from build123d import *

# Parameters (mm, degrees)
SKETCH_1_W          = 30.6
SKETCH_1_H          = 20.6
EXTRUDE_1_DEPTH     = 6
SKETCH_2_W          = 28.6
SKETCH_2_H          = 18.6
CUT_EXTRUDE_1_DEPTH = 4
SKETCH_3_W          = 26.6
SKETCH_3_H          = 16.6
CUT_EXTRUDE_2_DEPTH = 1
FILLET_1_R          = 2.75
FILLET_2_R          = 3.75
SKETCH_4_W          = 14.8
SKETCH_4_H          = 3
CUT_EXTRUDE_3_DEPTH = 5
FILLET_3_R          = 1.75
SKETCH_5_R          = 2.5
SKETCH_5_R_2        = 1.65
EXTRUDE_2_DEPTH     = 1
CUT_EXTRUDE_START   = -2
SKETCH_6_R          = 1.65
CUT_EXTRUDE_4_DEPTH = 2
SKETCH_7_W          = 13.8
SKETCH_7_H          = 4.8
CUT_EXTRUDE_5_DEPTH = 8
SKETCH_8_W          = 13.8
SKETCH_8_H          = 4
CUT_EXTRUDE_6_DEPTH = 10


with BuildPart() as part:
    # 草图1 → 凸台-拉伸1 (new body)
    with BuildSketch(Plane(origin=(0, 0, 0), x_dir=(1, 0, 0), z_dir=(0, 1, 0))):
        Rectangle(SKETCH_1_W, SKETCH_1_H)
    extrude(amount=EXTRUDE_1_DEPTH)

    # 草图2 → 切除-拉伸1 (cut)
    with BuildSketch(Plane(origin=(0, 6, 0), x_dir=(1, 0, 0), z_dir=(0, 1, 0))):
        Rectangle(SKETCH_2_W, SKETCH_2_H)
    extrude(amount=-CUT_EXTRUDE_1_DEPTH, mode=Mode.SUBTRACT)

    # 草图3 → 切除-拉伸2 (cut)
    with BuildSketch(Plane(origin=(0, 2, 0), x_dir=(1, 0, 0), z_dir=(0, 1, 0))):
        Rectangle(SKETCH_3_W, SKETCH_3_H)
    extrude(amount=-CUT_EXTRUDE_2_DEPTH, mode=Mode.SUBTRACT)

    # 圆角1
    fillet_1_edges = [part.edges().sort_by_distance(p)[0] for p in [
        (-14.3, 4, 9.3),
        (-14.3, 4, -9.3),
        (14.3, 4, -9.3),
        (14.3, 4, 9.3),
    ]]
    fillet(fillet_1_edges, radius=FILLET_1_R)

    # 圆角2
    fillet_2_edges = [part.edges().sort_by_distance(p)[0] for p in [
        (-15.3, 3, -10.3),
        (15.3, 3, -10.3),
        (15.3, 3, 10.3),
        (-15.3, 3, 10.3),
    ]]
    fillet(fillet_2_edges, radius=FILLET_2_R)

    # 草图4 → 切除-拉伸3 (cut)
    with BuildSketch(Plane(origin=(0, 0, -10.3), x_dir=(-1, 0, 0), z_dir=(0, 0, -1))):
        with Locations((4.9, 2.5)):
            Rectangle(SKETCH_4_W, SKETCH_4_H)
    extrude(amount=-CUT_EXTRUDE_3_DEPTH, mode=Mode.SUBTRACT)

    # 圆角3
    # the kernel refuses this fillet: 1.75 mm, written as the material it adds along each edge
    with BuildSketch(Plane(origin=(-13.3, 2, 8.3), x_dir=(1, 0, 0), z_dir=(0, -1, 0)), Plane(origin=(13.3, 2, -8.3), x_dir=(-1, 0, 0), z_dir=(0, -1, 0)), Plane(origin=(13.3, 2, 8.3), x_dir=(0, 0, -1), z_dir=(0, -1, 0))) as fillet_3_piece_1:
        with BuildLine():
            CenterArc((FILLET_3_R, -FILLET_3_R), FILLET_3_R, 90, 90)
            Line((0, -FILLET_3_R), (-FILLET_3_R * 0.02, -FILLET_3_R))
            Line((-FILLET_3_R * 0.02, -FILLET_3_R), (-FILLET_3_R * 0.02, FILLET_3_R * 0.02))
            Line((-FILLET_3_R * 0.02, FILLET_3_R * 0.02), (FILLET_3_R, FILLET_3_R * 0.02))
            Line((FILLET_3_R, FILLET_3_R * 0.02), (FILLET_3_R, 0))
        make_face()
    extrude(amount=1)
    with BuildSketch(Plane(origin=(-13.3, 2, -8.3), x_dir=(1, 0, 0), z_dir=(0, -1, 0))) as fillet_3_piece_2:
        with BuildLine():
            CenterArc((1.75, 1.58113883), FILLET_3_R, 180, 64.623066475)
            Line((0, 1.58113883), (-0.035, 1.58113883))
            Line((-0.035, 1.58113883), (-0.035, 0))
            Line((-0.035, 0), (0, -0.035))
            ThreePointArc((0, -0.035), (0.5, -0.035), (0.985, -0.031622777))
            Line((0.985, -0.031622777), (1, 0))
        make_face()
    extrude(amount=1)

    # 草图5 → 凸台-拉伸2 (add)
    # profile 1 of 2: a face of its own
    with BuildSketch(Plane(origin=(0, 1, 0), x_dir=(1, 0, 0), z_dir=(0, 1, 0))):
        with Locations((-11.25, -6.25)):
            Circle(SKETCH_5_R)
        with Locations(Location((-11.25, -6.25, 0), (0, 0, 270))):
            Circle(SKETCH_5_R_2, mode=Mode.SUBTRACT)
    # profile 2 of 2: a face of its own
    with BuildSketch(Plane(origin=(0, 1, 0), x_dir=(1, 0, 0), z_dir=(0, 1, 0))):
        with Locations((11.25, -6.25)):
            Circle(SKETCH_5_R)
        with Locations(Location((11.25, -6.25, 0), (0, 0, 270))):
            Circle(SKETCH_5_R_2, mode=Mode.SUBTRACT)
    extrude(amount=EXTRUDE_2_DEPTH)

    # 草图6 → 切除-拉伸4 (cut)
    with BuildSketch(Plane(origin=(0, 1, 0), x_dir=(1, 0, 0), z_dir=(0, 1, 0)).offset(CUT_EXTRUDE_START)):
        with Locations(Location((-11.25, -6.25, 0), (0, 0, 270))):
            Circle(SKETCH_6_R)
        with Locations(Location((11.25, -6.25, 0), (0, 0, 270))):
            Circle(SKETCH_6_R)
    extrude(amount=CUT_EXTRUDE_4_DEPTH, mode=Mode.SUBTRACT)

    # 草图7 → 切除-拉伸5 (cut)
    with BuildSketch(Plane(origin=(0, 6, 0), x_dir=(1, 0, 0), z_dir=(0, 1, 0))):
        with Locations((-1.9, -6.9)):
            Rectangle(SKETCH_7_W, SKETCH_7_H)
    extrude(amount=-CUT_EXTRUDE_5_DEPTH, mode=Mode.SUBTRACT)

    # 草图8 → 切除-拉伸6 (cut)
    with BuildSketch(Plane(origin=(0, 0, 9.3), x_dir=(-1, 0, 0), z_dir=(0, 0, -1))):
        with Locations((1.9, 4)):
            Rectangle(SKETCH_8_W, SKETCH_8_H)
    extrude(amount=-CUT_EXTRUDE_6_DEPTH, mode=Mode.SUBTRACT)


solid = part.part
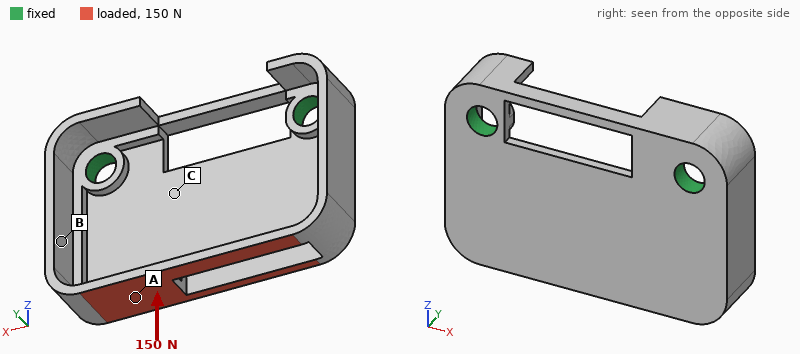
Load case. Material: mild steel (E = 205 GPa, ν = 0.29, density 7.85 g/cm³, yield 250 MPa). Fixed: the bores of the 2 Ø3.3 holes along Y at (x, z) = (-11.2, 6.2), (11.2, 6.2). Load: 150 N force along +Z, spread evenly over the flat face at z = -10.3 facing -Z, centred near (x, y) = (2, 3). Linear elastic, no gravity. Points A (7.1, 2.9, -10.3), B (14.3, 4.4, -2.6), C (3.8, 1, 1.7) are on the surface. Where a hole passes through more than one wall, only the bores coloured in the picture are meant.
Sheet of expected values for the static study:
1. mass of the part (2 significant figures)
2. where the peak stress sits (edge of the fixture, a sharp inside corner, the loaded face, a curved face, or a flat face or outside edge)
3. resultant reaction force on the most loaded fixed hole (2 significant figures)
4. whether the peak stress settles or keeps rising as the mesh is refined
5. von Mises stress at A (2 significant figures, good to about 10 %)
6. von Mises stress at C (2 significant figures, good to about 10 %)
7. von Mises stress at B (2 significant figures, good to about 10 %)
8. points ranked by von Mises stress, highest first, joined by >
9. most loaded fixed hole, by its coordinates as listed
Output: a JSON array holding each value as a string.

["7.7 g", "a sharp inside corner", "94 N", "keeps rising", "63 MPa", "14 MPa", "22 MPa", "A > B > C", "(11.2, 6.2)"]
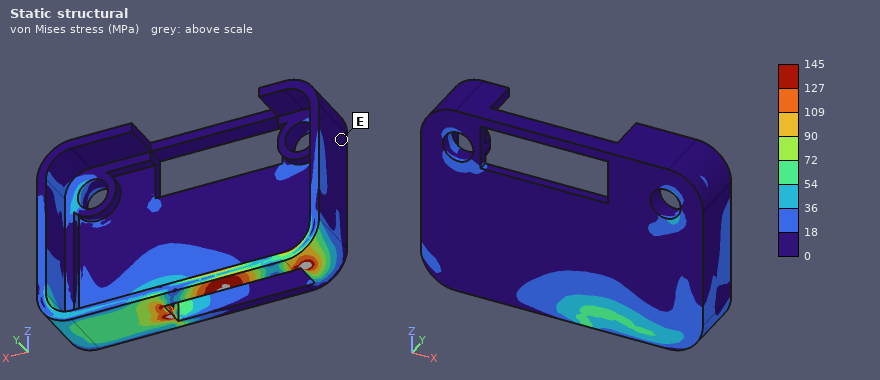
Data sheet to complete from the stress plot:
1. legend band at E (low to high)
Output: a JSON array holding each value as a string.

["0 to 18 MPa"]
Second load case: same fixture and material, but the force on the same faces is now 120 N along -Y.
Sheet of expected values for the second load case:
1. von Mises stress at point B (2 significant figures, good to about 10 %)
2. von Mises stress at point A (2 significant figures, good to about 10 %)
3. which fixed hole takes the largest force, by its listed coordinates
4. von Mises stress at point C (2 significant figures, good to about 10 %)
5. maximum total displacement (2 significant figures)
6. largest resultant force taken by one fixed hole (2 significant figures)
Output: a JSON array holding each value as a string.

["59 MPa", "34 MPa", "(11.2, 6.2)", "39 MPa", "64 µm", "81 N"]
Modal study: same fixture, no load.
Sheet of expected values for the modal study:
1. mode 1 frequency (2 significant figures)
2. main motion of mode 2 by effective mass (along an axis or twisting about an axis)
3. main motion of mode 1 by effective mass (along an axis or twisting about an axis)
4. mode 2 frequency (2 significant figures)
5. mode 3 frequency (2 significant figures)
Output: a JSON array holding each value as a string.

["5700 Hz", "twisting about Z", "along Y", "8800 Hz", "12 kHz"]
